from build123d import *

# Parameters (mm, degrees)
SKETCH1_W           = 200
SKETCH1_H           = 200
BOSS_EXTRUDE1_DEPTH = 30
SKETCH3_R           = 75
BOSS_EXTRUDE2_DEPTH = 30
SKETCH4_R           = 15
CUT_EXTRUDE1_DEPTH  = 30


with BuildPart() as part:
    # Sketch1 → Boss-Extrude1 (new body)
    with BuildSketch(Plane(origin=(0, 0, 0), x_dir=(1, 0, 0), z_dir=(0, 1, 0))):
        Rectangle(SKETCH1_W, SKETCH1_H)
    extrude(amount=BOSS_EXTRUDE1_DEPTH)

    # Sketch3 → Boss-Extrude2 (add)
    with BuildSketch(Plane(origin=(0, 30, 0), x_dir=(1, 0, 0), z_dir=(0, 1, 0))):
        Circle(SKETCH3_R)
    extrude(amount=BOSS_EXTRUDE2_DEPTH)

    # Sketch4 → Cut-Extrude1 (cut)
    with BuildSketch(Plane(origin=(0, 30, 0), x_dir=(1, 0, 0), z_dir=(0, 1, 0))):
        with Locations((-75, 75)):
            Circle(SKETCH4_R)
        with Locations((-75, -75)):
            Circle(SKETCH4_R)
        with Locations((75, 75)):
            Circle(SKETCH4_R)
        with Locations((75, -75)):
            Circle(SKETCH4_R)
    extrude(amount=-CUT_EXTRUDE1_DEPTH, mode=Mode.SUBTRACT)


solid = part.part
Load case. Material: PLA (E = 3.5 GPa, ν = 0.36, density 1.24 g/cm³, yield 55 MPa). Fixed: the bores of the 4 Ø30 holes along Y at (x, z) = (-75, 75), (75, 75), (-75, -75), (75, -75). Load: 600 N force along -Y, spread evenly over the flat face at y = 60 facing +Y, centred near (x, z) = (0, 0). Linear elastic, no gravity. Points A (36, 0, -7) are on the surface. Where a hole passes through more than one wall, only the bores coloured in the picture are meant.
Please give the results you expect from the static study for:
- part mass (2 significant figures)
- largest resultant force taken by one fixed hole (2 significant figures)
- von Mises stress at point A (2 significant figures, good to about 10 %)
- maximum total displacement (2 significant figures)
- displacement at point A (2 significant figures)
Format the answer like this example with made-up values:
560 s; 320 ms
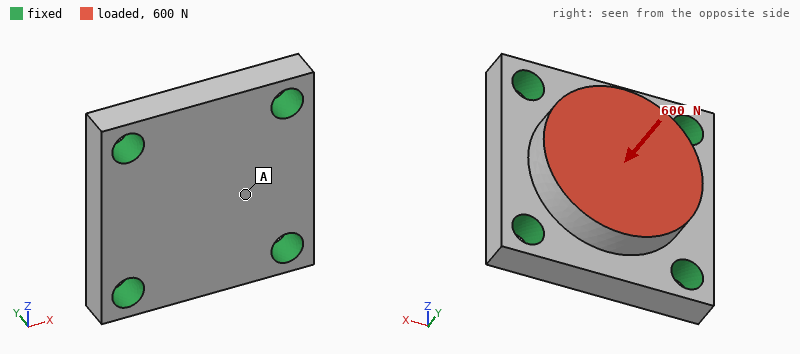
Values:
2.0 kg; 160 N; 0.063 MPa; 4.3 µm; 3.8 µm
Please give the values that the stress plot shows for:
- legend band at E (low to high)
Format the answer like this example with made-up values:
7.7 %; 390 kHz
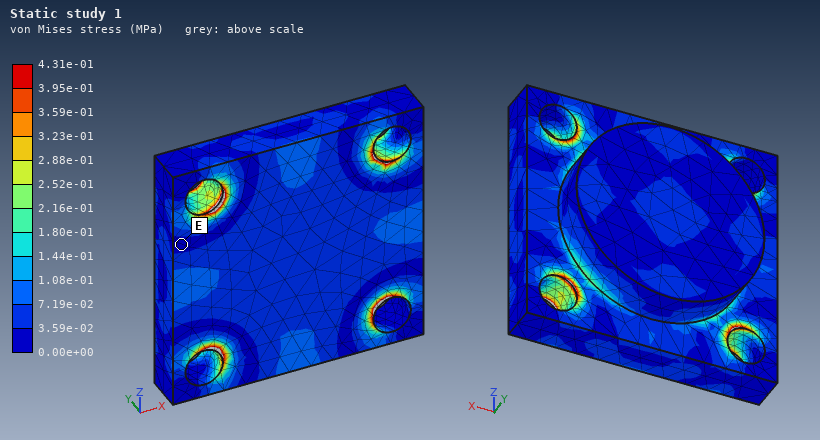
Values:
0.00e+00 to 3.59e-02 MPa
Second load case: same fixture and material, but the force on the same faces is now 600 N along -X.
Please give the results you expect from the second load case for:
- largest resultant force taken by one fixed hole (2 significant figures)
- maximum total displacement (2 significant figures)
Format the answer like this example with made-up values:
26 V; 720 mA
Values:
190 N; 5.0 µm
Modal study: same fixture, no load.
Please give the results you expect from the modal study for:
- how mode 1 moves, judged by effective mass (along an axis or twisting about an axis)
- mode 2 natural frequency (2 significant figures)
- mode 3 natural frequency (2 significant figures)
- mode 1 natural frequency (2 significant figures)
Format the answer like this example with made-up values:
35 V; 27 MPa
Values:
along Y; 2200 Hz; 2200 Hz; 1700 Hz
